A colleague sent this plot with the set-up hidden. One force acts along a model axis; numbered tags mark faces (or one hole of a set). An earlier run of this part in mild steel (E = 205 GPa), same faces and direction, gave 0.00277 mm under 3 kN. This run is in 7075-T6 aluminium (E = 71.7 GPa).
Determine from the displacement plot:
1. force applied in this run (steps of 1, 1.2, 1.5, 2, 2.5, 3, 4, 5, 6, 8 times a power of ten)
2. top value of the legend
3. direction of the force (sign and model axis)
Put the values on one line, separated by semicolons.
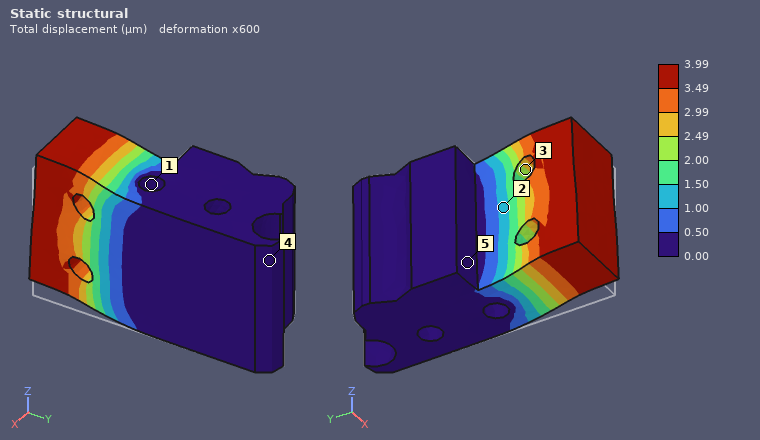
1.5 kN; 3.99 µm; +Z
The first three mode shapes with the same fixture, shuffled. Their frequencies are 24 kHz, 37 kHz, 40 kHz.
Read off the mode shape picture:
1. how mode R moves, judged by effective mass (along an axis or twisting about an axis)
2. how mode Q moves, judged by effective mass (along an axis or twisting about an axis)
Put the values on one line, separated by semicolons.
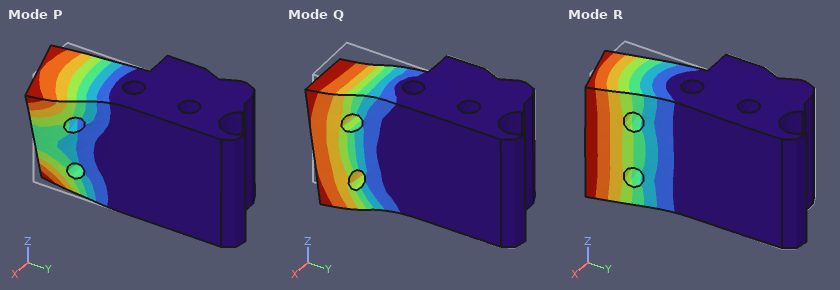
along X; along Z
